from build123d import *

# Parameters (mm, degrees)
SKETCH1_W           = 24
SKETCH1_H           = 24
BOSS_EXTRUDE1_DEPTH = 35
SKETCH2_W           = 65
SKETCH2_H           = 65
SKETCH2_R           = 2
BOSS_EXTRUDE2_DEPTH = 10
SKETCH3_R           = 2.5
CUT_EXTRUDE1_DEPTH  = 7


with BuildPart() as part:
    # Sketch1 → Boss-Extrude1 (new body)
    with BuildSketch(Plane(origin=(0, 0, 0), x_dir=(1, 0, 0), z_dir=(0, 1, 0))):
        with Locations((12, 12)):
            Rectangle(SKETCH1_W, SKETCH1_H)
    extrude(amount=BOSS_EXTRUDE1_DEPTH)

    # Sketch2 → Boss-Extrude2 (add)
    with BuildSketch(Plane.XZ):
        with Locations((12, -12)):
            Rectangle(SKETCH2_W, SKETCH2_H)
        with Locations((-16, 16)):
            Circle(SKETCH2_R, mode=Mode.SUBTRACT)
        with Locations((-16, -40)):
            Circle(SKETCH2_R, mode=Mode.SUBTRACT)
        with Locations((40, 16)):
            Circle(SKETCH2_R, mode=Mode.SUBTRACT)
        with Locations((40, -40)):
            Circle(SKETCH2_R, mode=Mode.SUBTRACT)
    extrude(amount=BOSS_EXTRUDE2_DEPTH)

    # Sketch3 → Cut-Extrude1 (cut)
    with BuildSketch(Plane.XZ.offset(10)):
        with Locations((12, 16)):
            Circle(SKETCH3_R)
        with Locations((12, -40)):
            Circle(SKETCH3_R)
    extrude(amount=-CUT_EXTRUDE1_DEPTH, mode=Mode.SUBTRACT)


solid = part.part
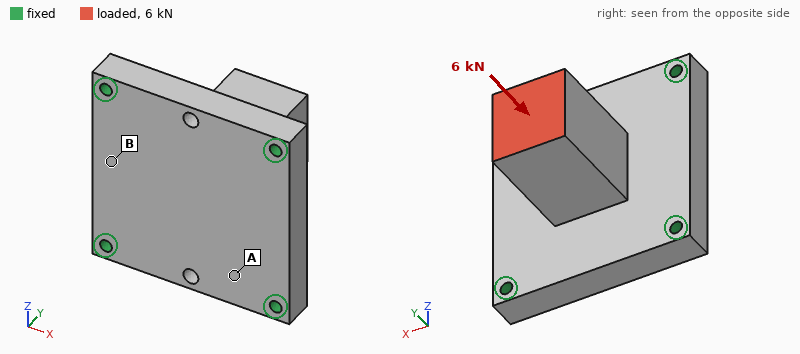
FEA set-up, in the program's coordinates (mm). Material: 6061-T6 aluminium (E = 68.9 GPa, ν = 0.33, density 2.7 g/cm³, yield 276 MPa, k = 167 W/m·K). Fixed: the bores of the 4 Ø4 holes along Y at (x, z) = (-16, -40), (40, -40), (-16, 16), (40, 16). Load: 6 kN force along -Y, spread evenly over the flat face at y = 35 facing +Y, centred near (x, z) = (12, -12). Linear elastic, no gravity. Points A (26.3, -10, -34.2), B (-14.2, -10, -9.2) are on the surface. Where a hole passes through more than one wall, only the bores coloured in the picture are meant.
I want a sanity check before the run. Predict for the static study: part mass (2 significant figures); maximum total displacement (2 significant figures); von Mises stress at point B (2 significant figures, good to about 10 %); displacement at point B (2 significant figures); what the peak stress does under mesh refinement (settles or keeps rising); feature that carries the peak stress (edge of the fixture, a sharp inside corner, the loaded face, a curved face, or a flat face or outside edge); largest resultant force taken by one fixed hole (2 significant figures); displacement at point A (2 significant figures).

170 g
38 µm
21 MPa
20 µm
keeps rising
edge of the fixture
1.5 kN
17 µm
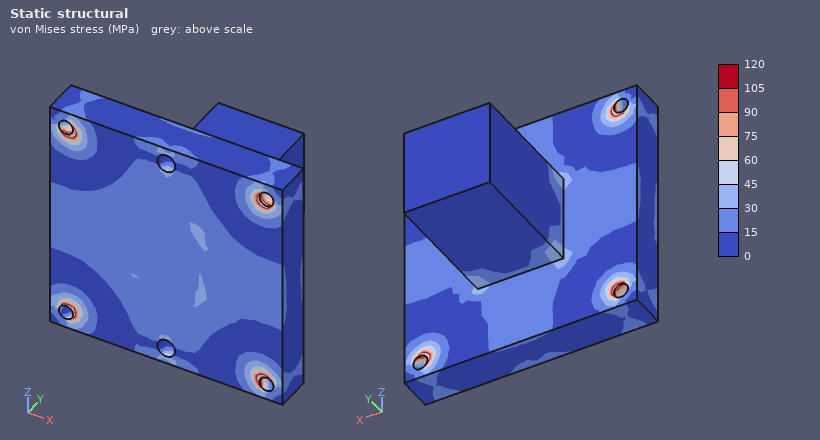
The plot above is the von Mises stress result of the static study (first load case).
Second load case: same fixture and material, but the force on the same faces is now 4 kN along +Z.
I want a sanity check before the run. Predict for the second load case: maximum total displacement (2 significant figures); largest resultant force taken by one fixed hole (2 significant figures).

0.12 mm
2.0 kN
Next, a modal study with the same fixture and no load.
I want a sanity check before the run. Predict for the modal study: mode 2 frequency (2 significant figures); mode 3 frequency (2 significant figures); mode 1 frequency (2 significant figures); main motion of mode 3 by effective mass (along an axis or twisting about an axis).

6300 Hz
6700 Hz
6300 Hz
along Y
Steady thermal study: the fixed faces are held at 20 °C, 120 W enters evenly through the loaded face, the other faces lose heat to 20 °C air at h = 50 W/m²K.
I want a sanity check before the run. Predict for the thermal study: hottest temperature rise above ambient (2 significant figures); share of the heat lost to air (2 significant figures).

66 K
11 %
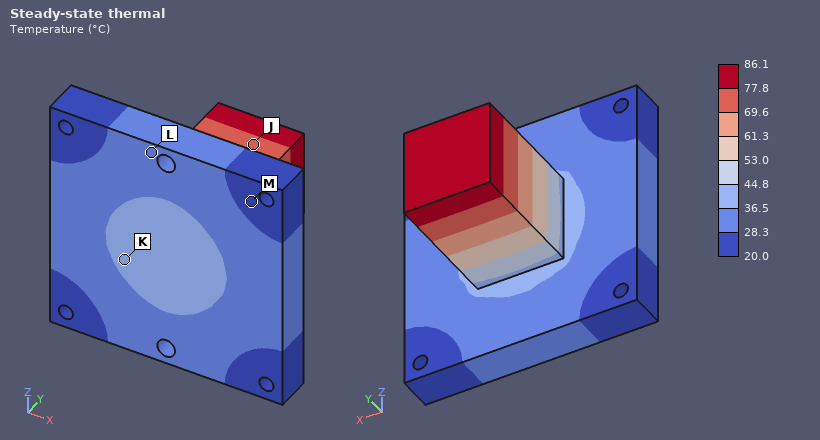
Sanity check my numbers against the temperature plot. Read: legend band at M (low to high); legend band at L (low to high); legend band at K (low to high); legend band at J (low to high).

20.0 to 28.3 °C
28.3 to 36.5 °C
36.5 to 44.8 °C
69.6 to 77.8 °C
